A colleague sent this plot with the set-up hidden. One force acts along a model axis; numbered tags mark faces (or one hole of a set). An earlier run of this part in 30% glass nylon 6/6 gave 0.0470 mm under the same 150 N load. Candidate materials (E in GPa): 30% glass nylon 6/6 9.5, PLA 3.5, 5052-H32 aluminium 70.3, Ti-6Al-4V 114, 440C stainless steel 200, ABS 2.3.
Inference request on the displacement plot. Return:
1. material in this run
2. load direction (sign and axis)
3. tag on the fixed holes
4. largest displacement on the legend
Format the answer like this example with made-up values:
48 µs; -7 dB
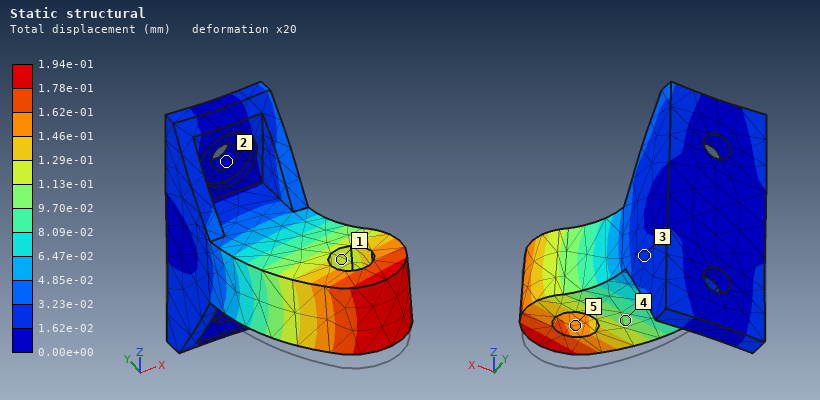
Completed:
ABS; +Z; 2; 1.94e-01 mm
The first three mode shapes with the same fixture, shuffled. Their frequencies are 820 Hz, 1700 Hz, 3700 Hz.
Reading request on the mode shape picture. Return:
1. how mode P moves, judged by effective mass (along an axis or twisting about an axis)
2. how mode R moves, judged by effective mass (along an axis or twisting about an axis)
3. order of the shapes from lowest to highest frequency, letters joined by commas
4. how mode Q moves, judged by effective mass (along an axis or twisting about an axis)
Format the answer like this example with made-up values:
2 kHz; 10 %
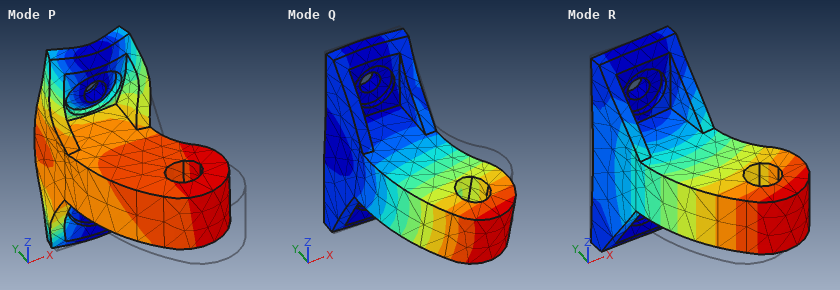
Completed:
along Y; along X; R, Q, P; along Z
